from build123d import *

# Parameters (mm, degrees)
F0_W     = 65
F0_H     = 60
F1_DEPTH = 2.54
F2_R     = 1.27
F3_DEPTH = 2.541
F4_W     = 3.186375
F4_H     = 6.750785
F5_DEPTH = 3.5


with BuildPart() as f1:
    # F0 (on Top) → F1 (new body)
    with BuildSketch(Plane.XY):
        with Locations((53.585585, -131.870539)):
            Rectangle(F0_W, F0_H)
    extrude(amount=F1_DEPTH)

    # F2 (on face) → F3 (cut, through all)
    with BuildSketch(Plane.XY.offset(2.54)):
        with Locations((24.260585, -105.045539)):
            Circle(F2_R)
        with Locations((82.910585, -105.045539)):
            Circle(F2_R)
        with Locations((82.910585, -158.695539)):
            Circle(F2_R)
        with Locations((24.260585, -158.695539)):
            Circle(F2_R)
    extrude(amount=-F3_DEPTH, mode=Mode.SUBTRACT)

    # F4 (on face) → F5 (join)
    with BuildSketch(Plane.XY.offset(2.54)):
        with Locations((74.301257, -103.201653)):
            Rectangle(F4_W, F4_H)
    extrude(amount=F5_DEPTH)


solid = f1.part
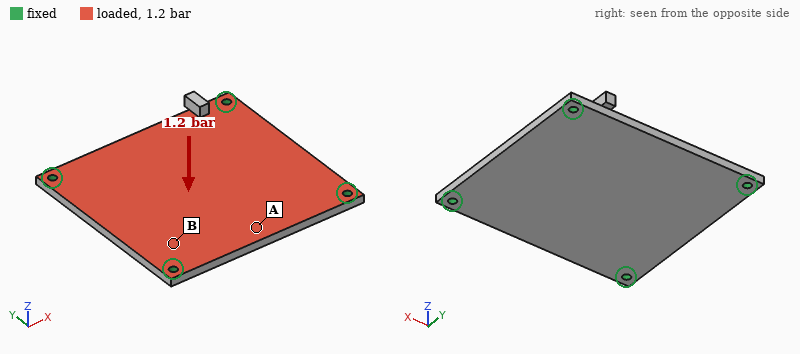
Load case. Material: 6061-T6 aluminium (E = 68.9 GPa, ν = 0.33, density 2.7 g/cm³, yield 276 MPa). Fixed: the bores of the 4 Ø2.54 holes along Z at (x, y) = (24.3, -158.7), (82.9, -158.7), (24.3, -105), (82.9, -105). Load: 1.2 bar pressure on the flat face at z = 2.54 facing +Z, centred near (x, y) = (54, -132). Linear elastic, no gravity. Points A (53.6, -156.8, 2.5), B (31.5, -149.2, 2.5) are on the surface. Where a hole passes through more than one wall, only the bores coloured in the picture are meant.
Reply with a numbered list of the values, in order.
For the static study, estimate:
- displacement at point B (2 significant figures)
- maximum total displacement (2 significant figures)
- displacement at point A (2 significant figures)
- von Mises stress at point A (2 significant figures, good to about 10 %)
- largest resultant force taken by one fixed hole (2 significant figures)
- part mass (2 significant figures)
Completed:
1. 37 µm
2. 100 µm
3. 68 µm
4. 23 MPa
5. 120 N
6. 27 g
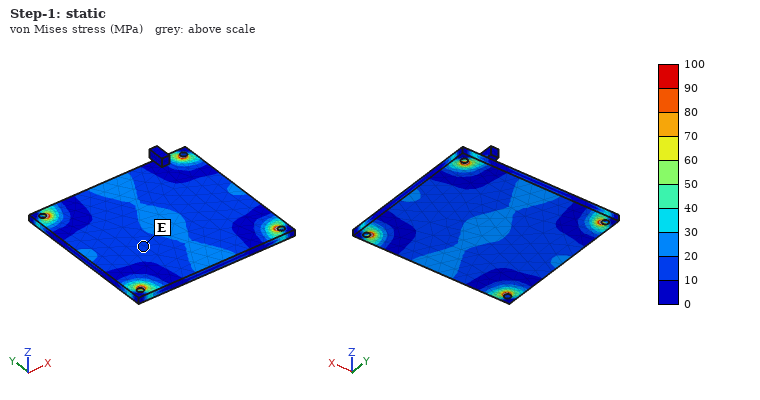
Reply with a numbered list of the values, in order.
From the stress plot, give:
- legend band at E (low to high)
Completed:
1. 10 to 20 MPa
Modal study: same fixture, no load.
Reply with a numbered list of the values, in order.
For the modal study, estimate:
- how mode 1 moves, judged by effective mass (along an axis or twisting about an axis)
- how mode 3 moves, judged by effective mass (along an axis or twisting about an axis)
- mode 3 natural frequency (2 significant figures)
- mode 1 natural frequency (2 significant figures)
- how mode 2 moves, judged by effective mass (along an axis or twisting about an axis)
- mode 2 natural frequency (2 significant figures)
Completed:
1. along Z
2. twisting about Y
3. 4700 Hz
4. 2500 Hz
5. twisting about X
6. 4300 Hz
